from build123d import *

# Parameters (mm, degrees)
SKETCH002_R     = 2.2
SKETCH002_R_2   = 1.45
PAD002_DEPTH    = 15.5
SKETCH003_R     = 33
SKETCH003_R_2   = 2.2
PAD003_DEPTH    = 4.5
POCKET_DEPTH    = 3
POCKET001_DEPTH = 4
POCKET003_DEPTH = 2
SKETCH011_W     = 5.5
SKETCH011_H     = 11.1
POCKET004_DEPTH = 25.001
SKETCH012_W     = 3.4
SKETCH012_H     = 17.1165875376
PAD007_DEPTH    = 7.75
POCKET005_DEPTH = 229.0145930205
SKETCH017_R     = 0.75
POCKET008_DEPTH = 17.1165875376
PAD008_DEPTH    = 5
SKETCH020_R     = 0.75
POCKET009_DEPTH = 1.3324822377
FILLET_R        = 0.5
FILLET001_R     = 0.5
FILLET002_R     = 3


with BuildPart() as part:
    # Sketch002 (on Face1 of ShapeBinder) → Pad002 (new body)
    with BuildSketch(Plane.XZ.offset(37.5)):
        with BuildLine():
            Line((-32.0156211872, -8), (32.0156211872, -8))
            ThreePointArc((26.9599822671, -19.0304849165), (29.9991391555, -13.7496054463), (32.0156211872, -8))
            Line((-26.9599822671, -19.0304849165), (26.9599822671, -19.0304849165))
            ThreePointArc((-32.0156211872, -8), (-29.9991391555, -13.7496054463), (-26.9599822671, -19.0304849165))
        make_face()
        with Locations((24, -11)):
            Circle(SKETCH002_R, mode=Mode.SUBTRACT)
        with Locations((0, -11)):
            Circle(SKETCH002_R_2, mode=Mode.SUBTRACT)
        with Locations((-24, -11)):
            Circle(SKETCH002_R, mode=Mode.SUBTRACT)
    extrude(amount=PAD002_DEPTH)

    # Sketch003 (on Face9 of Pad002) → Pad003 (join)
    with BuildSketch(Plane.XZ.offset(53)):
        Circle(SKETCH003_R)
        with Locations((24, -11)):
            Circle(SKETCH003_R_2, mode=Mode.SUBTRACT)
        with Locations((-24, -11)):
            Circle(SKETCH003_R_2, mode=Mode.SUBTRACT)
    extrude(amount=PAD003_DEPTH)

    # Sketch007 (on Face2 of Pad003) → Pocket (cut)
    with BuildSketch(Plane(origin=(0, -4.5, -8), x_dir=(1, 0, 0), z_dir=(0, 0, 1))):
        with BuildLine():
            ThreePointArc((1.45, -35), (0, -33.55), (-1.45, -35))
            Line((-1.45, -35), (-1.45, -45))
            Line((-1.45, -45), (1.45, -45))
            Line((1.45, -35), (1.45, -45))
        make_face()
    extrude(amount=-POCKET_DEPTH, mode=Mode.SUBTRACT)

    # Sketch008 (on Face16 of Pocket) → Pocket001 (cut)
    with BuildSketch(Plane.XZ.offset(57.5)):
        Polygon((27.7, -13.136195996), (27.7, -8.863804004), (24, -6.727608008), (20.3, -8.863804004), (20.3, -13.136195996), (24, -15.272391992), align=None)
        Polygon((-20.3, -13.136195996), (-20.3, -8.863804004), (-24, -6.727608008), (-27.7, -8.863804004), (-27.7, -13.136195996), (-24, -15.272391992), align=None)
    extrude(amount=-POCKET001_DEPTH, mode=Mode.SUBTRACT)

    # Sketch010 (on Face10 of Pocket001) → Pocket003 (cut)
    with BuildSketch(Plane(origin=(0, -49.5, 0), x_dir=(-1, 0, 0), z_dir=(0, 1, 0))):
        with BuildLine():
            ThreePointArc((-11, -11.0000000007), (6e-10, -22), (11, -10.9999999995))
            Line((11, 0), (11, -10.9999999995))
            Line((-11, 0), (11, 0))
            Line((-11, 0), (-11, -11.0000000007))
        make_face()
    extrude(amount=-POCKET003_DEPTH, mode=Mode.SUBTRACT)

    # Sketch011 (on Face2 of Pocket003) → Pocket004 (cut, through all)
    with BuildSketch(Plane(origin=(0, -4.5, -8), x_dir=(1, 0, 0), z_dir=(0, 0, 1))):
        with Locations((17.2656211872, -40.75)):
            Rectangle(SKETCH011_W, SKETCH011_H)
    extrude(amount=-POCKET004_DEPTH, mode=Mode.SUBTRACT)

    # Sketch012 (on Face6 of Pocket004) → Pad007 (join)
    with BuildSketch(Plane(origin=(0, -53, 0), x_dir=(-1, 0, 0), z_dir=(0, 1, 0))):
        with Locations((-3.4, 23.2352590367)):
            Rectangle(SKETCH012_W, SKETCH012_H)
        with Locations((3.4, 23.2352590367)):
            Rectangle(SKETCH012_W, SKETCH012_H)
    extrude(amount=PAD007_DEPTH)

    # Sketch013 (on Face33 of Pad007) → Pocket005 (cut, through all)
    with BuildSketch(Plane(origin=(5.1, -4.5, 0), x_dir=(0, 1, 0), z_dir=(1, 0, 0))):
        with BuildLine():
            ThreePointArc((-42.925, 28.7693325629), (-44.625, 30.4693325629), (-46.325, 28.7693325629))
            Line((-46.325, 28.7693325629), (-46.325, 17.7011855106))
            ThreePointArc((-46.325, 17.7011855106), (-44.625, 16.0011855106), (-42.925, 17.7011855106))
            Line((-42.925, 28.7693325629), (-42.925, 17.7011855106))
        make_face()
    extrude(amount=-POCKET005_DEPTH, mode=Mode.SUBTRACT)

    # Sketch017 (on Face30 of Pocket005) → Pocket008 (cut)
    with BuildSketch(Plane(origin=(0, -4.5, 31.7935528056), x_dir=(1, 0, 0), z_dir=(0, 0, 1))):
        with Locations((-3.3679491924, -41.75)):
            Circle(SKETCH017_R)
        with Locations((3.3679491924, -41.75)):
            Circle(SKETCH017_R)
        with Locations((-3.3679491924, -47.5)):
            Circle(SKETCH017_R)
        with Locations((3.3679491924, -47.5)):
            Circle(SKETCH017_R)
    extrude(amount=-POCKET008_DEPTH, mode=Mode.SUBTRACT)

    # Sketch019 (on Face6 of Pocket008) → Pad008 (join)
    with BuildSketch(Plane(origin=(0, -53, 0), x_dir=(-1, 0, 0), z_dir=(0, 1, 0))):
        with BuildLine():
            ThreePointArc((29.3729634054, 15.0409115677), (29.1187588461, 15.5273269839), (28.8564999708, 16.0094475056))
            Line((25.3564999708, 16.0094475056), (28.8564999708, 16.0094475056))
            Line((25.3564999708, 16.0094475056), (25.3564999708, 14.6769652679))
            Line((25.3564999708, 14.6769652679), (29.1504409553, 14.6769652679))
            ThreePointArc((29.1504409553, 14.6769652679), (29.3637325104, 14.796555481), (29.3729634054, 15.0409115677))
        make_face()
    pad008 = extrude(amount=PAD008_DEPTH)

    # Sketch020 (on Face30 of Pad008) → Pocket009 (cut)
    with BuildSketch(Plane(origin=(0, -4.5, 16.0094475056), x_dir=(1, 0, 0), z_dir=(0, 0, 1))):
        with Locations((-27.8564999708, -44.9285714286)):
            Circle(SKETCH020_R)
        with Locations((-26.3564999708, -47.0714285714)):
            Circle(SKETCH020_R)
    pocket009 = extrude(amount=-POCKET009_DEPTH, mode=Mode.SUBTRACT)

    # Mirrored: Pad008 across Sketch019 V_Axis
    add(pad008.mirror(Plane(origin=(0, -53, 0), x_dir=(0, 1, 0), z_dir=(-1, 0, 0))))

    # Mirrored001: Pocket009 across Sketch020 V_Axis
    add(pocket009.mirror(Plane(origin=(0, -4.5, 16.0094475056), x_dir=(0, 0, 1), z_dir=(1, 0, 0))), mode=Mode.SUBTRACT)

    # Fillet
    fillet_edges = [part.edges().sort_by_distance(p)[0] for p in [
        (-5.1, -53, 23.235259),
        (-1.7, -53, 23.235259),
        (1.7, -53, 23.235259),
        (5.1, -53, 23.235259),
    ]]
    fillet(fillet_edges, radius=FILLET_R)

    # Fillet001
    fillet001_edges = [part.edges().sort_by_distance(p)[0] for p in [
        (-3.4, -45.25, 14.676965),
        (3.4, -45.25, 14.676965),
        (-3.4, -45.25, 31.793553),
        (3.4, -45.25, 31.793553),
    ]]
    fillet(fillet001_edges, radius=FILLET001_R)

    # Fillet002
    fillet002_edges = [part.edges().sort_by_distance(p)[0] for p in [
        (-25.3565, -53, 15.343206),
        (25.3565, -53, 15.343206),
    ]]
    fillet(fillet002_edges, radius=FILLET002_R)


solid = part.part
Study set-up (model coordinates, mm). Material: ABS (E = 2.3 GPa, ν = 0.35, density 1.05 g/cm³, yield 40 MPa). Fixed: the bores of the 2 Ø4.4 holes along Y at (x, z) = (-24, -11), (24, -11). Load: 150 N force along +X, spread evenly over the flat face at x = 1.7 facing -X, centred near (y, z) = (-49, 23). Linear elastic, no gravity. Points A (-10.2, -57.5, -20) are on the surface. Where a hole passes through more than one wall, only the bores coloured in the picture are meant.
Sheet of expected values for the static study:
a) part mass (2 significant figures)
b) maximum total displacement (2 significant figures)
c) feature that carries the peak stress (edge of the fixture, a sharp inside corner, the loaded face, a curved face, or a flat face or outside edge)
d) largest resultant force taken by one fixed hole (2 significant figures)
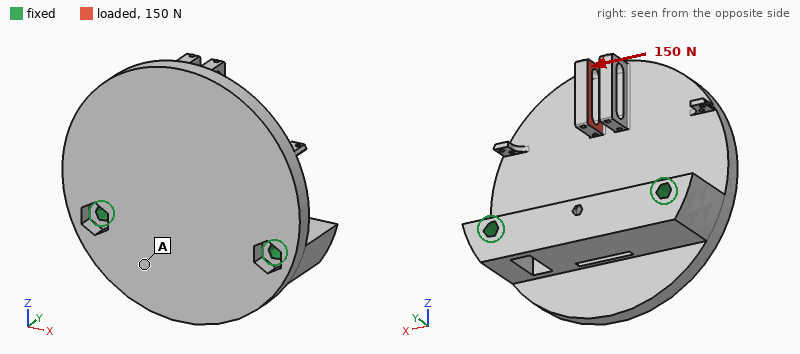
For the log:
25 g
0.94 mm
the loaded face
130 N
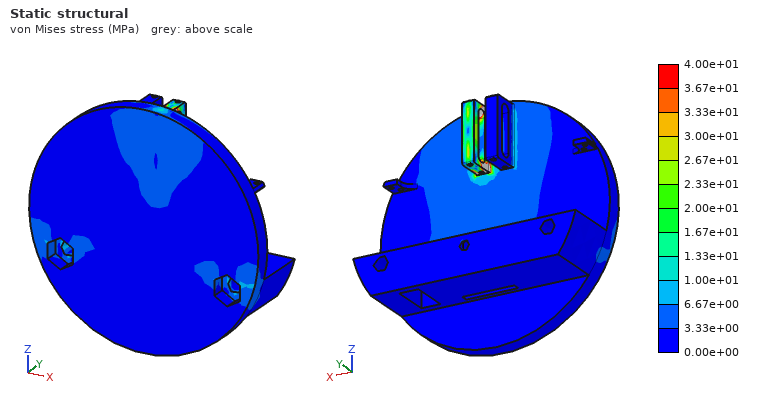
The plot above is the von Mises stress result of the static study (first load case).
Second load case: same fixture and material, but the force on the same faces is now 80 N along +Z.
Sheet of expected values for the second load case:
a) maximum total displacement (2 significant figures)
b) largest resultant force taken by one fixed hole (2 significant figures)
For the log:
0.57 mm
43 N
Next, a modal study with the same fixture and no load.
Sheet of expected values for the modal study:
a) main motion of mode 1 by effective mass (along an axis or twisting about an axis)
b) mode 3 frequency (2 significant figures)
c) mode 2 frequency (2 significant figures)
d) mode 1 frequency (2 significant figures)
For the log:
along Y
2700 Hz
1500 Hz
600 Hz
